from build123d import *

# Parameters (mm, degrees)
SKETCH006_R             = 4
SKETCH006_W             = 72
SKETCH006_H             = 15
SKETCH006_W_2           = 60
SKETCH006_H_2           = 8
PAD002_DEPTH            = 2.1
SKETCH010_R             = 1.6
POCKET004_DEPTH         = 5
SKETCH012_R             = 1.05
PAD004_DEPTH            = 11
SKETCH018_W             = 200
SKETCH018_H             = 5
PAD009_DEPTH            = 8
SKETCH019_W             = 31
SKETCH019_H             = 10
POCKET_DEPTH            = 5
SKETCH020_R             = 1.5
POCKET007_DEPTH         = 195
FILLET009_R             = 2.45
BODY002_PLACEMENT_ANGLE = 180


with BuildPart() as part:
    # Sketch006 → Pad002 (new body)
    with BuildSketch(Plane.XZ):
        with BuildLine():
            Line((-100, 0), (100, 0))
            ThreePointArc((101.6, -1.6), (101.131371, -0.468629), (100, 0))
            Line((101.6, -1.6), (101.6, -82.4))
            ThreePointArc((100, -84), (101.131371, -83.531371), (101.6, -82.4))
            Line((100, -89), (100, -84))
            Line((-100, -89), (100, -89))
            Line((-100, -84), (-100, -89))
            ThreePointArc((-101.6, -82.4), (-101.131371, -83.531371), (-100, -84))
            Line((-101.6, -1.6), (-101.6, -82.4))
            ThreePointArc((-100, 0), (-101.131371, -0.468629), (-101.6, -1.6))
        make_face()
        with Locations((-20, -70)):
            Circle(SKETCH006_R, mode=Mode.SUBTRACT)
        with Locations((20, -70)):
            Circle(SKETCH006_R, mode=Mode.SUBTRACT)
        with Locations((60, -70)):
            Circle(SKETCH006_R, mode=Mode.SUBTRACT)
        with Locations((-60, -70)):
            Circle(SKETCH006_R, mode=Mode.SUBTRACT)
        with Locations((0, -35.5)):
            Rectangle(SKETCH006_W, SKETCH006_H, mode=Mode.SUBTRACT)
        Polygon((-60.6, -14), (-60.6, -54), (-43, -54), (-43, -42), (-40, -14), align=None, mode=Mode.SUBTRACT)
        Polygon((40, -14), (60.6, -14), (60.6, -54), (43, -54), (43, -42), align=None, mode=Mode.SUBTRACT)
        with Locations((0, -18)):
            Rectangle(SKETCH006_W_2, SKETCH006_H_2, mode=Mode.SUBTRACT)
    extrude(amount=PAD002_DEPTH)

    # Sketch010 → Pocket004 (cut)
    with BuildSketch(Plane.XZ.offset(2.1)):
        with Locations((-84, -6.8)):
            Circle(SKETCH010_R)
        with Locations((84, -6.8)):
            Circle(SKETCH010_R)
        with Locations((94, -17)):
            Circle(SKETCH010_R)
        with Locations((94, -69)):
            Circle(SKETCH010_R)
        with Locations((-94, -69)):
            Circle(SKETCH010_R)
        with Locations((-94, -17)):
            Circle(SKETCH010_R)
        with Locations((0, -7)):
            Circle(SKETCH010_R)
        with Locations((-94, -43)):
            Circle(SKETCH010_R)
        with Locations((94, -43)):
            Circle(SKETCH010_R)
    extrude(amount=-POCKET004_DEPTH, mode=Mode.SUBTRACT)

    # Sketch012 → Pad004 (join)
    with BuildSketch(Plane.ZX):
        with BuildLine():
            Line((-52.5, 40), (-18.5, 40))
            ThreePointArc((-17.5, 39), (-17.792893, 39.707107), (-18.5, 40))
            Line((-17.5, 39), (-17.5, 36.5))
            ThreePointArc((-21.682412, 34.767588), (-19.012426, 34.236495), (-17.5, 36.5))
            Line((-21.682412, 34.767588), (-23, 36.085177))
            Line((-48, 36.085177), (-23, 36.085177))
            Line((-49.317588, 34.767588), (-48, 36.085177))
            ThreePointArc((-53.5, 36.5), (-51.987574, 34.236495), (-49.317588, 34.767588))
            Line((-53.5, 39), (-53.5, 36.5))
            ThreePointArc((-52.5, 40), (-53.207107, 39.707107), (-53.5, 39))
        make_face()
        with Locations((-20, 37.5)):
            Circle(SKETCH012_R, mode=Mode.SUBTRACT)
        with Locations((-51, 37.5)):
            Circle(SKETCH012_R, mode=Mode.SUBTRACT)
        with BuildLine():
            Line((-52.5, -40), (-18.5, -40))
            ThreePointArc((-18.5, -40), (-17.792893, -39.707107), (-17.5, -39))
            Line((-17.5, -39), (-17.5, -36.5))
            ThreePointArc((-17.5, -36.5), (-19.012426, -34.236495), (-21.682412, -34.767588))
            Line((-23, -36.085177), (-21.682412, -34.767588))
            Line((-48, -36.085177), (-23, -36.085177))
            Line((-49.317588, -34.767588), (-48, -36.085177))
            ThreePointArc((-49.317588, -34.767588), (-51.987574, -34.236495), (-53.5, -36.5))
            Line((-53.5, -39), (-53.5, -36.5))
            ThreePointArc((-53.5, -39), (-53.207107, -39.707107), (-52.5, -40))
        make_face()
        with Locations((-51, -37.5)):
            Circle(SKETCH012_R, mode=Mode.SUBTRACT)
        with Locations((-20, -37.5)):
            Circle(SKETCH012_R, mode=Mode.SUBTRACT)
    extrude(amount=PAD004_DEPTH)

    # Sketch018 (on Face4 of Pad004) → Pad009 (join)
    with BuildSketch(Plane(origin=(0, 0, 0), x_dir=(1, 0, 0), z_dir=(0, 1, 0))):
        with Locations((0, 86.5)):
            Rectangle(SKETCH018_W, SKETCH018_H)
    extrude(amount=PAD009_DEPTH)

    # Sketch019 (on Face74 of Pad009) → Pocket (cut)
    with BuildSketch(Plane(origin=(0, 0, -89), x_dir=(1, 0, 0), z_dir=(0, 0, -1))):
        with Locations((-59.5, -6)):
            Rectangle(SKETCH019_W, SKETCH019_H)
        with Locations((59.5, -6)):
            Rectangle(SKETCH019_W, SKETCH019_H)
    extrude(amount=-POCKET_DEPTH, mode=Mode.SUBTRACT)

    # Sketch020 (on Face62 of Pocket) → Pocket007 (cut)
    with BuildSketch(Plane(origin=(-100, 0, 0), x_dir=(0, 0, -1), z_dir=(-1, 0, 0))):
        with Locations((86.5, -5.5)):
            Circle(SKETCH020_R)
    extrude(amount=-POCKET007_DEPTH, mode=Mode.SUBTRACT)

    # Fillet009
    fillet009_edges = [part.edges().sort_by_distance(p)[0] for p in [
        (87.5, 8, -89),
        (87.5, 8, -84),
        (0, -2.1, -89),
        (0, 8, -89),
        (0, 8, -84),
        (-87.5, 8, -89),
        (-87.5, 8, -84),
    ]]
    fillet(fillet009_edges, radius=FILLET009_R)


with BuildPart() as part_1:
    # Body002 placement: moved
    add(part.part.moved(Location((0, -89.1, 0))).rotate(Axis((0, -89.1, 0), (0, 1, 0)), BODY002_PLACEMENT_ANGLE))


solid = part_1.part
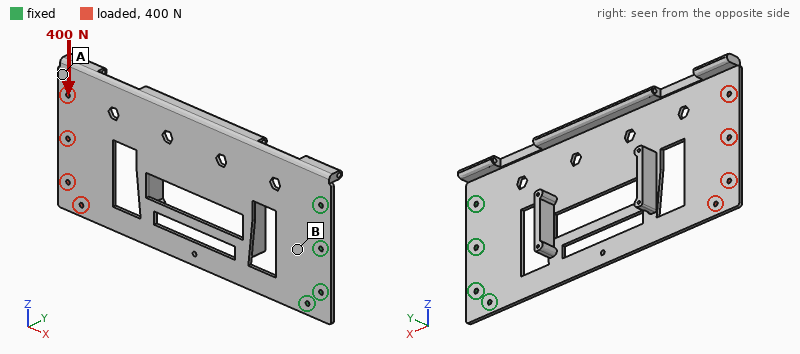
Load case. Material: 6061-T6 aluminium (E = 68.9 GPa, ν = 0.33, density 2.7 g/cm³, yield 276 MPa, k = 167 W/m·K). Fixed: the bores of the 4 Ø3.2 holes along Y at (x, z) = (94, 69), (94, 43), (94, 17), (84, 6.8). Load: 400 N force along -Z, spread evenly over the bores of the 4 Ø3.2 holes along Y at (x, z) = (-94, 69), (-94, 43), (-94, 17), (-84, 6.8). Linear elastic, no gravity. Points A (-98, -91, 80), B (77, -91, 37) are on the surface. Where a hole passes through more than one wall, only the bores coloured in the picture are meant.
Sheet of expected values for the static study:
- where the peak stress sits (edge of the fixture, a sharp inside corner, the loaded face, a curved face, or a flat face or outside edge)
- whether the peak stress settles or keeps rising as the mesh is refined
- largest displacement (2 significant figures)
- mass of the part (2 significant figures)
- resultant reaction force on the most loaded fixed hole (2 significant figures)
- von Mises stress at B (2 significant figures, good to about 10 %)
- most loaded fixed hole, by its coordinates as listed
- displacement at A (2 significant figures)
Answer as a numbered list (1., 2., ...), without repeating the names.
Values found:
1. edge of the fixture
2. keeps rising
3. 0.75 mm
4. 100 g
5. 1.2 kN
6. 17 MPa
7. (94, 69)
8. 0.73 mm
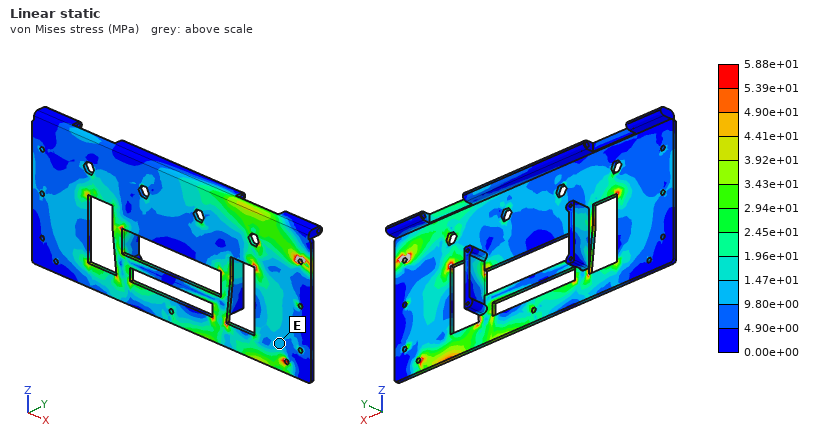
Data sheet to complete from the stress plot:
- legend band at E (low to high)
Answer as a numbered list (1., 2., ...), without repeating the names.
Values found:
1. 9.80e+00 to 1.47e+01 MPa
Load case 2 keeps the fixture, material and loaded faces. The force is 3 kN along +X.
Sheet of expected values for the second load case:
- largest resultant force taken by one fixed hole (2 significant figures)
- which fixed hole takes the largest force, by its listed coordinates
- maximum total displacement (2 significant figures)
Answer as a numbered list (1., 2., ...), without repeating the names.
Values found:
1. 1.2 kN
2. (84, 6.8)
3. 0.29 mm
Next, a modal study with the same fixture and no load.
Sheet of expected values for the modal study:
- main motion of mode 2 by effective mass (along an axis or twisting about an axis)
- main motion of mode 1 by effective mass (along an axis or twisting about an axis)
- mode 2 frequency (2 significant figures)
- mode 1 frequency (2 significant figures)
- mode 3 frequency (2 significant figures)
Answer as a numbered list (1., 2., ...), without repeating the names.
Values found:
1. twisting about X
2. along Y
3. 210 Hz
4. 47 Hz
5. 360 Hz
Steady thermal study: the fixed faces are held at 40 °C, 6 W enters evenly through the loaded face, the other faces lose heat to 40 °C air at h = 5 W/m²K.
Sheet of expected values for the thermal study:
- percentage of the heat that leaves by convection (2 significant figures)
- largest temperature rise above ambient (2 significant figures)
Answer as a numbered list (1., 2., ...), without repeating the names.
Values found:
1. 47 %
2. 36 K
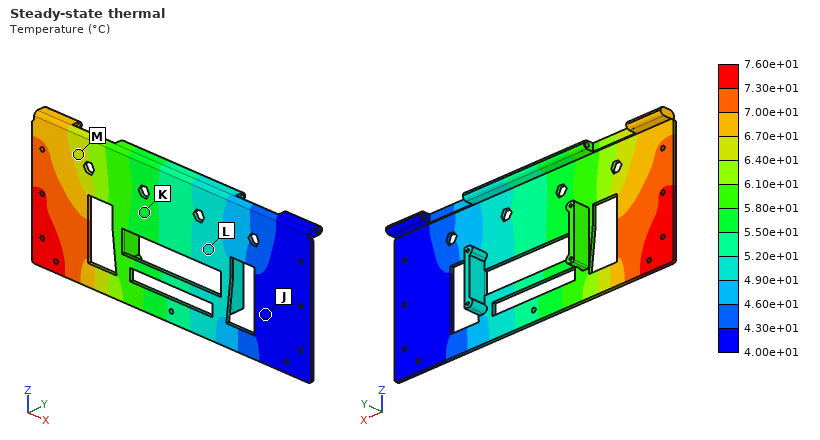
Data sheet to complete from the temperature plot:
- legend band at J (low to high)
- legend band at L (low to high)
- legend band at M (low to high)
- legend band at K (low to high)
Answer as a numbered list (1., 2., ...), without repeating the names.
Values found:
1. 4.00e+01 to 4.30e+01 °C
2. 4.90e+01 to 5.20e+01 °C
3. 6.40e+01 to 6.70e+01 °C
4. 5.50e+01 to 5.80e+01 °C
